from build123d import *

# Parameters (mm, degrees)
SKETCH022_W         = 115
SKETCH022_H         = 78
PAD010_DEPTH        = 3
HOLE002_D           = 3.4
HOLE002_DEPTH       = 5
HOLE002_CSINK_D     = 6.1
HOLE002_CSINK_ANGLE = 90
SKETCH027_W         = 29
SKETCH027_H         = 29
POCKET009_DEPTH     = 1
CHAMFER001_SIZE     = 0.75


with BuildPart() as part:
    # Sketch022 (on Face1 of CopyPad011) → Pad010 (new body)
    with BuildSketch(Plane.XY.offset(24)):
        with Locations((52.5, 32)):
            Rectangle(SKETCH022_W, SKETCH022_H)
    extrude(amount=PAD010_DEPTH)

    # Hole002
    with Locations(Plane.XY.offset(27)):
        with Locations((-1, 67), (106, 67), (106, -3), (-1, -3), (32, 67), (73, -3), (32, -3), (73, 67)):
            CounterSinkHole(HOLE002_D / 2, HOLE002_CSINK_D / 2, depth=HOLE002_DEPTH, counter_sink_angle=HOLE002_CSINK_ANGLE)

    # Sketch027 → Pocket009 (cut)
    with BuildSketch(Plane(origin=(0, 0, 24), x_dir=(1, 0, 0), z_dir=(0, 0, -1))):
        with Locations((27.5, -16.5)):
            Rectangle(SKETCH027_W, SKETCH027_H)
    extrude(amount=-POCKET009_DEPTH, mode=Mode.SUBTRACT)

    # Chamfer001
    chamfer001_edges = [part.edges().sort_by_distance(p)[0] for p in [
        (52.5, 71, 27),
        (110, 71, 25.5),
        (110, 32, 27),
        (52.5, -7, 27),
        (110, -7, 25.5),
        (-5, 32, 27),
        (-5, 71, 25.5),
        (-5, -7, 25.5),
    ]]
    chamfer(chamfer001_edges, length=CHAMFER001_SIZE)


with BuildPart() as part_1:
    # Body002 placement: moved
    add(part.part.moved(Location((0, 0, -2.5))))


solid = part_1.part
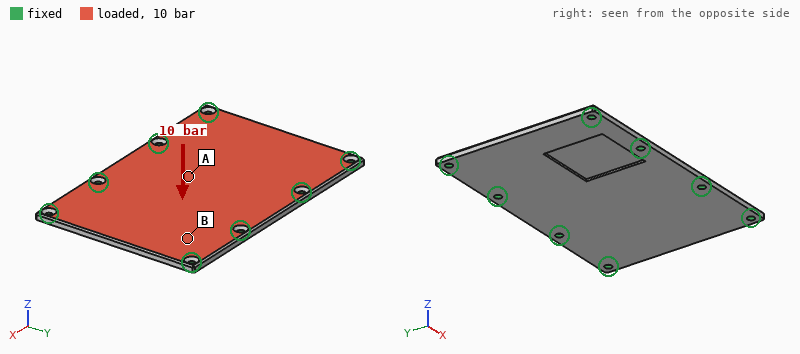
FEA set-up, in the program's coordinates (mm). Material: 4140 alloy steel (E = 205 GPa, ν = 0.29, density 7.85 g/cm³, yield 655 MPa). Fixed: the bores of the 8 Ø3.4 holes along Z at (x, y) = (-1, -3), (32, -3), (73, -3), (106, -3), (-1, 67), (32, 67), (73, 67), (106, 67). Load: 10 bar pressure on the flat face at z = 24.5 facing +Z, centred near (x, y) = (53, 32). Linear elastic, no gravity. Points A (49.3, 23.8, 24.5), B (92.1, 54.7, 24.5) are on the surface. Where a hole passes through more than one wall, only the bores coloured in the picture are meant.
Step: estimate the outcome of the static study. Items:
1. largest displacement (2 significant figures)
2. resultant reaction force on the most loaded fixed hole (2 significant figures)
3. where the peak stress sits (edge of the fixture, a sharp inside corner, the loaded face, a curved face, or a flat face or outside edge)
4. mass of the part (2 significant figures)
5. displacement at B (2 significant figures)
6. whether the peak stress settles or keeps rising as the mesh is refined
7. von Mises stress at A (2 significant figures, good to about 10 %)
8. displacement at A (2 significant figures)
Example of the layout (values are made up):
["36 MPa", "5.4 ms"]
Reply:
["0.27 mm", "2.1 kN", "edge of the fixture", "200 g", "0.10 mm", "keeps rising", "170 MPa", "0.25 mm"]
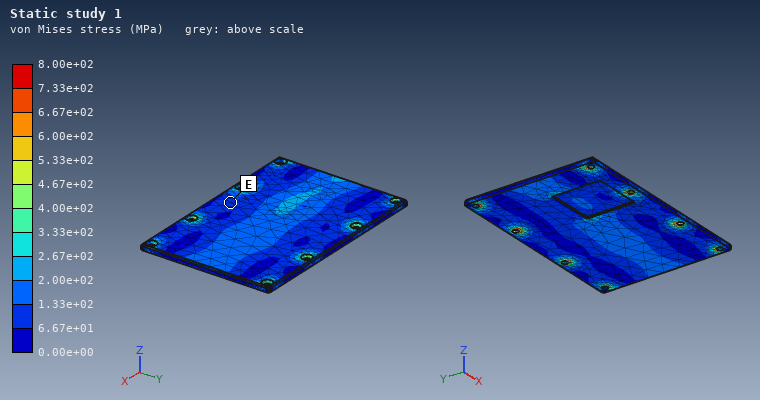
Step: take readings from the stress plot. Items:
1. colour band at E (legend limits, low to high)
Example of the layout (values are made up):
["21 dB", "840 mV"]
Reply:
["6.67e+01 to 1.33e+02 MPa"]
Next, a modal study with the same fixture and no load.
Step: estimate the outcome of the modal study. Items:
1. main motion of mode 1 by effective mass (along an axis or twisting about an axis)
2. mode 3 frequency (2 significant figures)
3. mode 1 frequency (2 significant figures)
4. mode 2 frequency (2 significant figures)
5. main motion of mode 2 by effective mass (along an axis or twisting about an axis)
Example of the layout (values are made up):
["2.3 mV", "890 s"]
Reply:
["along Z", "3700 Hz", "2400 Hz", "2900 Hz", "twisting about Y"]
